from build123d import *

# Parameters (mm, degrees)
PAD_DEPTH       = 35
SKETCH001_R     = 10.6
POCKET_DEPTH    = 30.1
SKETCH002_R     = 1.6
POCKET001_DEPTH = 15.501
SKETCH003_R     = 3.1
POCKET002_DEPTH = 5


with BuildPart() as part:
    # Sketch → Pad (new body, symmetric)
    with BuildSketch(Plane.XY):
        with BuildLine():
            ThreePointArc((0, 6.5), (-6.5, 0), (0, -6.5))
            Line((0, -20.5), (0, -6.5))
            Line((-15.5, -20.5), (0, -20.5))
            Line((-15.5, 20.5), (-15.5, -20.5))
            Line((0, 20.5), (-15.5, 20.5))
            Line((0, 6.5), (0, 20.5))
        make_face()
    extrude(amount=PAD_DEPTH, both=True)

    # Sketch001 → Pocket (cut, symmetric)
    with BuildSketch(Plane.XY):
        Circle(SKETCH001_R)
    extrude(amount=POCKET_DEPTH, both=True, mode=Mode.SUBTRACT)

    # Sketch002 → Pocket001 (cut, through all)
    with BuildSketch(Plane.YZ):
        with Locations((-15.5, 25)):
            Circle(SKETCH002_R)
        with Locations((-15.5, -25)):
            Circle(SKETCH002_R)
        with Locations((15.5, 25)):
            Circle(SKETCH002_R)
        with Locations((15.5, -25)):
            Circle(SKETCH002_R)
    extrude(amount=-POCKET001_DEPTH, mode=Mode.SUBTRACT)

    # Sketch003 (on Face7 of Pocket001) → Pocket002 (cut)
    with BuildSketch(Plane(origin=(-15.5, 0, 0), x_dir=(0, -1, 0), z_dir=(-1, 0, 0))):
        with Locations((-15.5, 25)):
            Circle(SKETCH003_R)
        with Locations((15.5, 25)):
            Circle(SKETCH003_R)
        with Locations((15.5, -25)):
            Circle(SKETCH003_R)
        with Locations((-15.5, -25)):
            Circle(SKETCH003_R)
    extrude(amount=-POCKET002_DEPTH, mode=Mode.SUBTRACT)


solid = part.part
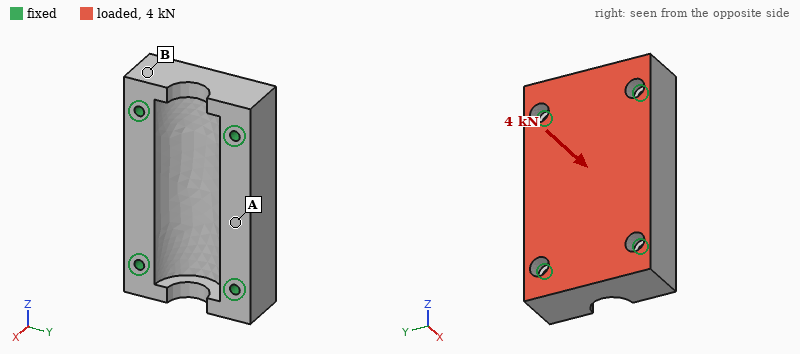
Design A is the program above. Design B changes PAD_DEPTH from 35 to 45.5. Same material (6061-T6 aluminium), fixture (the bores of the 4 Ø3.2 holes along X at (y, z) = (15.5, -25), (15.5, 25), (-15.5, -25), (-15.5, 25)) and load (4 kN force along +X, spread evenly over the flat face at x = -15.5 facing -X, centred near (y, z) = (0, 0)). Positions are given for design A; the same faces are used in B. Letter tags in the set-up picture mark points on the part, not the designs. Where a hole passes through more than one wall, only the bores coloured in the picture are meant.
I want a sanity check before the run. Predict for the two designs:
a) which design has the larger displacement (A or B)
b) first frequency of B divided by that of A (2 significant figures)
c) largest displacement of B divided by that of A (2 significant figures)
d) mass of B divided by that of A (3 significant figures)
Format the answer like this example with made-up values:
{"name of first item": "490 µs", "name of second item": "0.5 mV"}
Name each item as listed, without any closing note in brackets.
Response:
{"which design has the larger displacement": "A", "first frequency of B divided by that of A": "0.82", "largest displacement of B divided by that of A": "0.67", "mass of B divided by that of A": "1.37"}
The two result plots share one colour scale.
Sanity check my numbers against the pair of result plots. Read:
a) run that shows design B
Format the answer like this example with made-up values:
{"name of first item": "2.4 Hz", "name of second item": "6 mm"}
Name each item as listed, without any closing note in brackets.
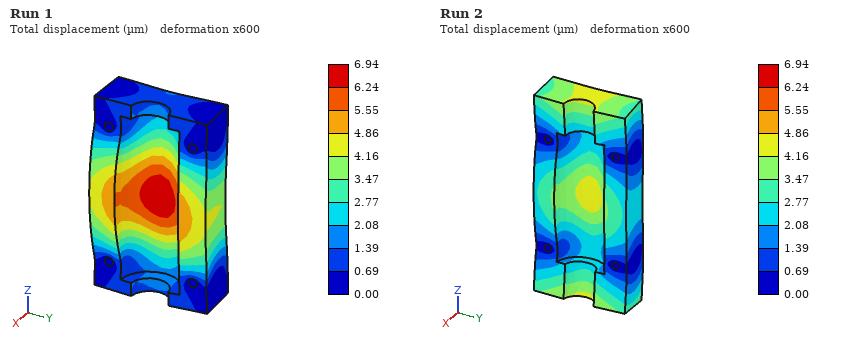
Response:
{"run that shows design B": "Run 2"}
